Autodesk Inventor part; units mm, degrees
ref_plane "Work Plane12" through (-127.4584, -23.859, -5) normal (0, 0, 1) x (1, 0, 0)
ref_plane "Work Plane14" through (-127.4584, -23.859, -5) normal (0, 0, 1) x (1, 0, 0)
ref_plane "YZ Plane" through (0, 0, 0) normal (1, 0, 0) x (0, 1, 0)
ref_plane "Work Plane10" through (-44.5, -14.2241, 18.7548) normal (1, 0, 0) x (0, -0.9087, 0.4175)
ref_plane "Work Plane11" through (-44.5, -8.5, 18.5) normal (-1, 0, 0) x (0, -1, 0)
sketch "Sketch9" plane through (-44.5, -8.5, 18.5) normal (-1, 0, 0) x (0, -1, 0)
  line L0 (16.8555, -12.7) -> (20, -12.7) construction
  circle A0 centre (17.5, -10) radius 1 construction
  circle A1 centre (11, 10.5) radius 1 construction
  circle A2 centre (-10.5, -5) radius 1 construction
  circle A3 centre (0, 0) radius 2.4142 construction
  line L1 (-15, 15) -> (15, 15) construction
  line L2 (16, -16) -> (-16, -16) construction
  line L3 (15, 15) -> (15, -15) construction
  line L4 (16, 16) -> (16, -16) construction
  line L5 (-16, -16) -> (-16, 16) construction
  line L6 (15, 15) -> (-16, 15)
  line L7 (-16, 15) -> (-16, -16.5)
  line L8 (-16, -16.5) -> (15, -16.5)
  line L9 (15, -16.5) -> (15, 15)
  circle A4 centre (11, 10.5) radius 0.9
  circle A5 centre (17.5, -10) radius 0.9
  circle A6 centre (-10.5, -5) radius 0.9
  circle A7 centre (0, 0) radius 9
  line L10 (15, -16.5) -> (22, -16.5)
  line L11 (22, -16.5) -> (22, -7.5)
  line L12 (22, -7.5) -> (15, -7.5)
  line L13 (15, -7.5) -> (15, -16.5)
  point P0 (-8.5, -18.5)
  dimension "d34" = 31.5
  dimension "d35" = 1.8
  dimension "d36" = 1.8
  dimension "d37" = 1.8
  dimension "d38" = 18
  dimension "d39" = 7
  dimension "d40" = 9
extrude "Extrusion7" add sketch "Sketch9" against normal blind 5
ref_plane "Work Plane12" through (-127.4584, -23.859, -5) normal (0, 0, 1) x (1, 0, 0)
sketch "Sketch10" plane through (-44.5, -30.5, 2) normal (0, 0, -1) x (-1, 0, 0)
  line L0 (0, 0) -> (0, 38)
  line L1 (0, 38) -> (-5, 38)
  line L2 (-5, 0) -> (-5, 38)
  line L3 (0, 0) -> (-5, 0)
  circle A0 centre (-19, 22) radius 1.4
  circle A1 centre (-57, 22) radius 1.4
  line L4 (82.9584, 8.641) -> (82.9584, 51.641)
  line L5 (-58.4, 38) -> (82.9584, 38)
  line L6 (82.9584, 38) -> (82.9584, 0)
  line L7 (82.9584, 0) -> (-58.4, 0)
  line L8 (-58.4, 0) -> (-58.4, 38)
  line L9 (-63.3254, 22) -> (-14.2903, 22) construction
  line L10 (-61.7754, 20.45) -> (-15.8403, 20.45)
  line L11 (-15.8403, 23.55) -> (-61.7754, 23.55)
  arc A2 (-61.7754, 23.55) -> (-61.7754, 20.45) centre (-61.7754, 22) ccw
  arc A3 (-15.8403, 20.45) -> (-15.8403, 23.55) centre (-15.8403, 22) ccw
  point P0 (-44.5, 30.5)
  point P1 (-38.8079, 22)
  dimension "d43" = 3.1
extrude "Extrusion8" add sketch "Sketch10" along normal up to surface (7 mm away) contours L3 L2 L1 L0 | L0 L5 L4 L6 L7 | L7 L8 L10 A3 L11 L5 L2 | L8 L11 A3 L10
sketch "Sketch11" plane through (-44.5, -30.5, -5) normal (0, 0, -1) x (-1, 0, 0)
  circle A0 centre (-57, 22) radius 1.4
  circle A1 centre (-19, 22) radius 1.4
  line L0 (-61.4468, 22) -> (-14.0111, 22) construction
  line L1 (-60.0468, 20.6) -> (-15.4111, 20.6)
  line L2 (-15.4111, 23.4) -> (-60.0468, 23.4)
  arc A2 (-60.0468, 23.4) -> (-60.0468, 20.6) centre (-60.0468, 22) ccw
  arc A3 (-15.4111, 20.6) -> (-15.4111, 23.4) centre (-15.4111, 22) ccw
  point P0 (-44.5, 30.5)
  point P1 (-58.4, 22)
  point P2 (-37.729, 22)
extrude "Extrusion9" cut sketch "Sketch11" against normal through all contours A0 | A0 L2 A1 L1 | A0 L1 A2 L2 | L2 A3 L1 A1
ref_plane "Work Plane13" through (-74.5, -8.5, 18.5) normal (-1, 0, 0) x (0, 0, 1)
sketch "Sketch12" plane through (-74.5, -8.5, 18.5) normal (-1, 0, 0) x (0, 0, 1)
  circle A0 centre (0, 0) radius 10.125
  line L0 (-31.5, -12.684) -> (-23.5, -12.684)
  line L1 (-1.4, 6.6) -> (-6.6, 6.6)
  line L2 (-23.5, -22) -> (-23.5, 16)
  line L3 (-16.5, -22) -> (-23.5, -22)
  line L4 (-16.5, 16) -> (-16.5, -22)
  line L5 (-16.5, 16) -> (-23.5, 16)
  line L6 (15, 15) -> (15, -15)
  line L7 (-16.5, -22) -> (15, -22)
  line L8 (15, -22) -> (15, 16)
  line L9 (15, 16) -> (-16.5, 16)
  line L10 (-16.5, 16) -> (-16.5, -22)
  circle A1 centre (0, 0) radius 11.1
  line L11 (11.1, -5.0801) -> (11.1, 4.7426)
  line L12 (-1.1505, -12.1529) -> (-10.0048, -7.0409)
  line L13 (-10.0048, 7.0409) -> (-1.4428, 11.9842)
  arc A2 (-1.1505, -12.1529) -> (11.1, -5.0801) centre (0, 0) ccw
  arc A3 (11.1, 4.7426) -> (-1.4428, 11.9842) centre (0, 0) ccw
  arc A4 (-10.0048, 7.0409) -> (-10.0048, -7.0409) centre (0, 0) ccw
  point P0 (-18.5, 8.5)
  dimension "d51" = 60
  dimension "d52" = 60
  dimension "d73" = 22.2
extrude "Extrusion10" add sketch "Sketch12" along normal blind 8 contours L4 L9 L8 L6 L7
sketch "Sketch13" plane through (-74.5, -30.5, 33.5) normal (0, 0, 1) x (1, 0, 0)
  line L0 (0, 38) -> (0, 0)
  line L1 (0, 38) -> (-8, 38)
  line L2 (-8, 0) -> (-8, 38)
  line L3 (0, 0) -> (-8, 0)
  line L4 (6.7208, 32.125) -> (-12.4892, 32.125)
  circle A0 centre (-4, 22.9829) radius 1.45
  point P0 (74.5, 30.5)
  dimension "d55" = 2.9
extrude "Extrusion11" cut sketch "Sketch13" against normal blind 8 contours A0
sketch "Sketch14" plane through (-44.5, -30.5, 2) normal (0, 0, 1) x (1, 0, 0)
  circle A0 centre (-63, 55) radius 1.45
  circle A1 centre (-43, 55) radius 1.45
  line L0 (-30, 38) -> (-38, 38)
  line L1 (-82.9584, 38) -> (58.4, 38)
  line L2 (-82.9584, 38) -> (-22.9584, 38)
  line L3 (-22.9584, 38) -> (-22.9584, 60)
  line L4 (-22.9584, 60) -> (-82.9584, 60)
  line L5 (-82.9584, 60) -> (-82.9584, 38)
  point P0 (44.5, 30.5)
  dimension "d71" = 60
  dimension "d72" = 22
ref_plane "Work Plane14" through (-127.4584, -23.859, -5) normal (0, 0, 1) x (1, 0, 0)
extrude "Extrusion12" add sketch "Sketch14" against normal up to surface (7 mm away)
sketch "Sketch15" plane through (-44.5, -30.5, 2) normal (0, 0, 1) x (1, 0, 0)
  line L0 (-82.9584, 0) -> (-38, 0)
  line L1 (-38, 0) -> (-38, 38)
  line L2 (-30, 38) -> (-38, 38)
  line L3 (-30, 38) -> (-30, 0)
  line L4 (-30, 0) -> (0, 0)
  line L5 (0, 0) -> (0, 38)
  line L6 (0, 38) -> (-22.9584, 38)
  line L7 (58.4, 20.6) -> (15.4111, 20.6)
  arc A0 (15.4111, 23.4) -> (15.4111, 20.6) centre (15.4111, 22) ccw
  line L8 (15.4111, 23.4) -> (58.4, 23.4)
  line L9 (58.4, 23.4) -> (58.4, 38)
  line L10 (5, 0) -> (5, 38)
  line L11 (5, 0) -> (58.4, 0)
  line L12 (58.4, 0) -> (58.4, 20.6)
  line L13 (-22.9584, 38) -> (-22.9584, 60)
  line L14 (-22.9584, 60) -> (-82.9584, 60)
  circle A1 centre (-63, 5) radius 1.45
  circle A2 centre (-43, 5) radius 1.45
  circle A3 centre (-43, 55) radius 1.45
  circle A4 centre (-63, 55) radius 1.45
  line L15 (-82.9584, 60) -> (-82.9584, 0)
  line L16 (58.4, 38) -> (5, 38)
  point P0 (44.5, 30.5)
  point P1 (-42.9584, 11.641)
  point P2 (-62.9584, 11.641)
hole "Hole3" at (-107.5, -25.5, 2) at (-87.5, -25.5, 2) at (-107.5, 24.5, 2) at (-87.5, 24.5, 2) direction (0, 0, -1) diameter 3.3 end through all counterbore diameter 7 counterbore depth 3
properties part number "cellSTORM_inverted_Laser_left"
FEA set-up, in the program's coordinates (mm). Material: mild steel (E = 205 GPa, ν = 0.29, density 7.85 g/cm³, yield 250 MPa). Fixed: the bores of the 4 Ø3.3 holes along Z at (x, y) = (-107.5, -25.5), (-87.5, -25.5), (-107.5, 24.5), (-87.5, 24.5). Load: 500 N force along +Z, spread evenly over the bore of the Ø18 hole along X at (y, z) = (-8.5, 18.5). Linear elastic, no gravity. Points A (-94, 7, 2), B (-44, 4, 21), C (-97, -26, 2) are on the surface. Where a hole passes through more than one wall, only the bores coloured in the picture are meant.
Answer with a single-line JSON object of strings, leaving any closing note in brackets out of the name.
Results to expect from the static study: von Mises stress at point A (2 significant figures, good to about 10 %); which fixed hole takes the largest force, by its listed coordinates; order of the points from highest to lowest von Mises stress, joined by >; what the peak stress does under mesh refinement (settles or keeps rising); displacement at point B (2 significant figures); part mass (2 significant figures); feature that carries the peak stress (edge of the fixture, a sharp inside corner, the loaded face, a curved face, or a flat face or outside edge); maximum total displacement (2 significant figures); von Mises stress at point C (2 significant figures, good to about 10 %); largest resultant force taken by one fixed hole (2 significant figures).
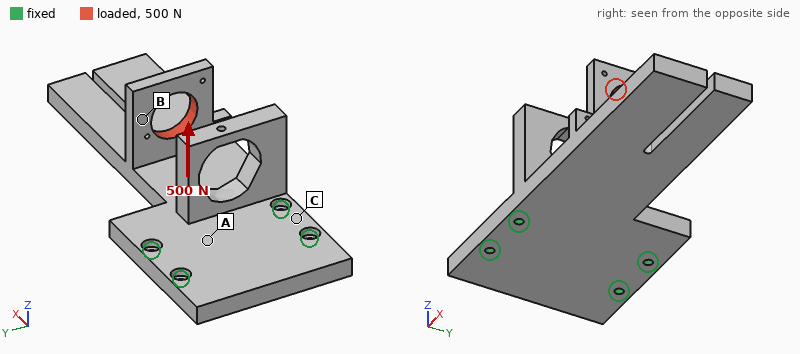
{"von Mises stress at point A": "23 MPa", "which fixed hole takes the largest force, by its listed coordinates": "(-87.5, -25.5)", "order of the points from highest to lowest von Mises stress, joined by >": "A > C > B", "what the peak stress does under mesh refinement": "keeps rising", "displacement at point B": "0.092 mm", "part mass": "430 g", "feature that carries the peak stress": "edge of the fixture", "maximum total displacement": "0.21 mm", "von Mises stress at point C": "15 MPa", "largest resultant force taken by one fixed hole": "980 N"}
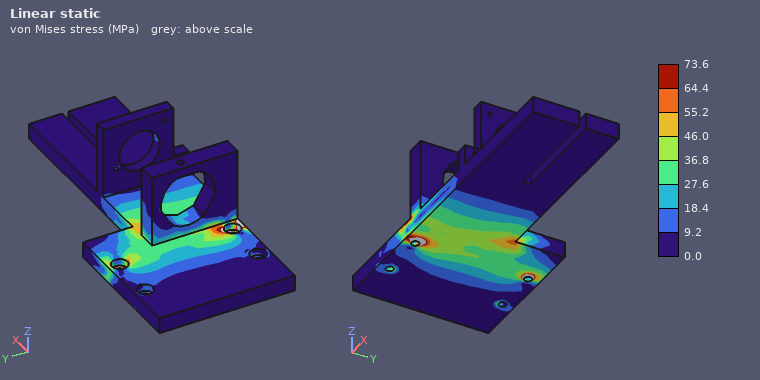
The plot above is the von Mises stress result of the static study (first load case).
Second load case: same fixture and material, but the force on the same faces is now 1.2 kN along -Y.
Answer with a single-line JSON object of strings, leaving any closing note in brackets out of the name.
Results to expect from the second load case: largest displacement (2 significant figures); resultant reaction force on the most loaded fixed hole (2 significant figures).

{"largest displacement": "0.10 mm", "resultant reaction force on the most loaded fixed hole": "1.3 kN"}
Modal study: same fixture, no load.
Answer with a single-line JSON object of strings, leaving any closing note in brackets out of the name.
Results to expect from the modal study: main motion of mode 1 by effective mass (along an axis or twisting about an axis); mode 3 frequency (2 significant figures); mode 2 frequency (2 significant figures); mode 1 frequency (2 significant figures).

{"main motion of mode 1 by effective mass": "along Z", "mode 3 frequency": "2700 Hz", "mode 2 frequency": "1800 Hz", "mode 1 frequency": "550 Hz"}
